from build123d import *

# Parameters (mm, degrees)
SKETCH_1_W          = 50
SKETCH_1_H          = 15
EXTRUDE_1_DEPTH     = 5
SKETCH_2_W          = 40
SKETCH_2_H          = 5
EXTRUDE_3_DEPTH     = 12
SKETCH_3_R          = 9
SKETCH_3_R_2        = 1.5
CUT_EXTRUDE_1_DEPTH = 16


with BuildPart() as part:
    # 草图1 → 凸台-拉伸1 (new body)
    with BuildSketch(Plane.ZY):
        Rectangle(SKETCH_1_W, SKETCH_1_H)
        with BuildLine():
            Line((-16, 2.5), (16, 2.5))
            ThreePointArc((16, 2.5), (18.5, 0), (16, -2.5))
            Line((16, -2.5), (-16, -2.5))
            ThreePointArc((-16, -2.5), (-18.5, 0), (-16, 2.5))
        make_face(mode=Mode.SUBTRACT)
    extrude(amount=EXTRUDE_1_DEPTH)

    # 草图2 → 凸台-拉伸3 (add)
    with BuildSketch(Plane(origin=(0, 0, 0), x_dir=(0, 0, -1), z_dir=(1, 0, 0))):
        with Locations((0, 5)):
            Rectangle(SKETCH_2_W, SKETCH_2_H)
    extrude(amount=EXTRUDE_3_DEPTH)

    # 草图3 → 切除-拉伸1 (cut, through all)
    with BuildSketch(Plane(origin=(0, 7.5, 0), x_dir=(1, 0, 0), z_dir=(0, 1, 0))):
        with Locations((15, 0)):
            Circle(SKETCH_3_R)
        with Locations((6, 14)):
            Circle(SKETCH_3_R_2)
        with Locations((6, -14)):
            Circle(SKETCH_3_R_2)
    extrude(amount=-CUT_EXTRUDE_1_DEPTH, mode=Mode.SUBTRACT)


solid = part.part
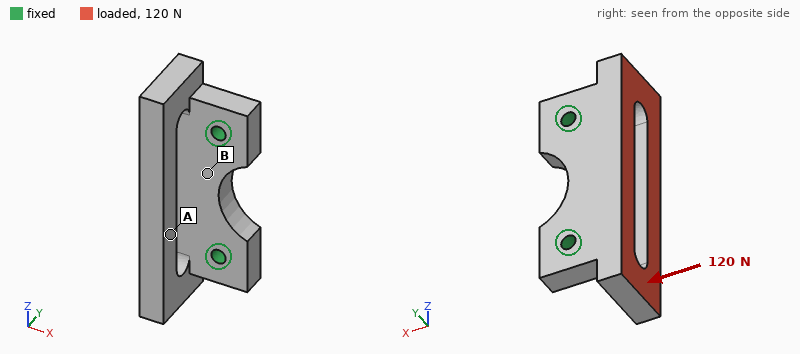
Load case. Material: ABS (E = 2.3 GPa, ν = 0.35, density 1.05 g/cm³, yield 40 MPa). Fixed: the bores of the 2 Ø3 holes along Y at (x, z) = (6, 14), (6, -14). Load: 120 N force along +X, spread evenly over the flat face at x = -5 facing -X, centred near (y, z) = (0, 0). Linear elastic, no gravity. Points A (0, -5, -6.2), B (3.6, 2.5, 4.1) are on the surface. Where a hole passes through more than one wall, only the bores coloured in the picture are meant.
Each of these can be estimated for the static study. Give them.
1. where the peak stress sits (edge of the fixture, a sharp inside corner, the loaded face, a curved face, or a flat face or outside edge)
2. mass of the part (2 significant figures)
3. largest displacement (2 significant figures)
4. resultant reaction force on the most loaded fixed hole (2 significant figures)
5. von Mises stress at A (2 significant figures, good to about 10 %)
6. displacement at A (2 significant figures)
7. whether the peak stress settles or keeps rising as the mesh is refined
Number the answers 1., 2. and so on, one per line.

1. a sharp inside corner
2. 5.1 g
3. 0.38 mm
4. 60 N
5. 4.2 MPa
6. 0.30 mm
7. keeps rising
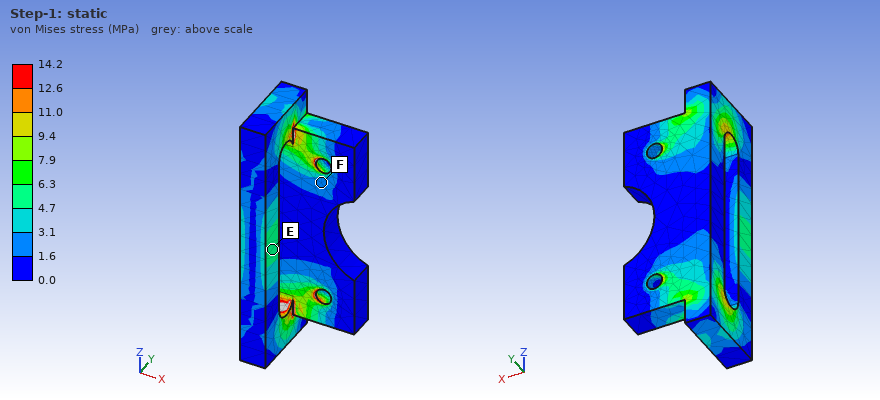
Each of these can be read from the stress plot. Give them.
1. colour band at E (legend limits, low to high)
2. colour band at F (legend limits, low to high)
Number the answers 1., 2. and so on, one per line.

1. 4.7 to 6.3 MPa
2. 1.6 to 3.1 MPa
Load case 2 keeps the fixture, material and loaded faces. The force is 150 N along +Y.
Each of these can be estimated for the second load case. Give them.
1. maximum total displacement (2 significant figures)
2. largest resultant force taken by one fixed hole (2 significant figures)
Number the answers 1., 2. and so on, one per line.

1. 0.39 mm
2. 75 N
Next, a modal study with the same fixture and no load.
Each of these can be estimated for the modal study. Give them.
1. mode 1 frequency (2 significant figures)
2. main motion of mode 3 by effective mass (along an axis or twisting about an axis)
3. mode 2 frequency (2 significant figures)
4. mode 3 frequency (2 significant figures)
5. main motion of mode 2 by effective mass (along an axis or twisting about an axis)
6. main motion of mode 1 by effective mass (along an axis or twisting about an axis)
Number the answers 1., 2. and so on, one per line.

1. 1900 Hz
2. along Y
3. 2800 Hz
4. 3300 Hz
5. along Z
6. along X
